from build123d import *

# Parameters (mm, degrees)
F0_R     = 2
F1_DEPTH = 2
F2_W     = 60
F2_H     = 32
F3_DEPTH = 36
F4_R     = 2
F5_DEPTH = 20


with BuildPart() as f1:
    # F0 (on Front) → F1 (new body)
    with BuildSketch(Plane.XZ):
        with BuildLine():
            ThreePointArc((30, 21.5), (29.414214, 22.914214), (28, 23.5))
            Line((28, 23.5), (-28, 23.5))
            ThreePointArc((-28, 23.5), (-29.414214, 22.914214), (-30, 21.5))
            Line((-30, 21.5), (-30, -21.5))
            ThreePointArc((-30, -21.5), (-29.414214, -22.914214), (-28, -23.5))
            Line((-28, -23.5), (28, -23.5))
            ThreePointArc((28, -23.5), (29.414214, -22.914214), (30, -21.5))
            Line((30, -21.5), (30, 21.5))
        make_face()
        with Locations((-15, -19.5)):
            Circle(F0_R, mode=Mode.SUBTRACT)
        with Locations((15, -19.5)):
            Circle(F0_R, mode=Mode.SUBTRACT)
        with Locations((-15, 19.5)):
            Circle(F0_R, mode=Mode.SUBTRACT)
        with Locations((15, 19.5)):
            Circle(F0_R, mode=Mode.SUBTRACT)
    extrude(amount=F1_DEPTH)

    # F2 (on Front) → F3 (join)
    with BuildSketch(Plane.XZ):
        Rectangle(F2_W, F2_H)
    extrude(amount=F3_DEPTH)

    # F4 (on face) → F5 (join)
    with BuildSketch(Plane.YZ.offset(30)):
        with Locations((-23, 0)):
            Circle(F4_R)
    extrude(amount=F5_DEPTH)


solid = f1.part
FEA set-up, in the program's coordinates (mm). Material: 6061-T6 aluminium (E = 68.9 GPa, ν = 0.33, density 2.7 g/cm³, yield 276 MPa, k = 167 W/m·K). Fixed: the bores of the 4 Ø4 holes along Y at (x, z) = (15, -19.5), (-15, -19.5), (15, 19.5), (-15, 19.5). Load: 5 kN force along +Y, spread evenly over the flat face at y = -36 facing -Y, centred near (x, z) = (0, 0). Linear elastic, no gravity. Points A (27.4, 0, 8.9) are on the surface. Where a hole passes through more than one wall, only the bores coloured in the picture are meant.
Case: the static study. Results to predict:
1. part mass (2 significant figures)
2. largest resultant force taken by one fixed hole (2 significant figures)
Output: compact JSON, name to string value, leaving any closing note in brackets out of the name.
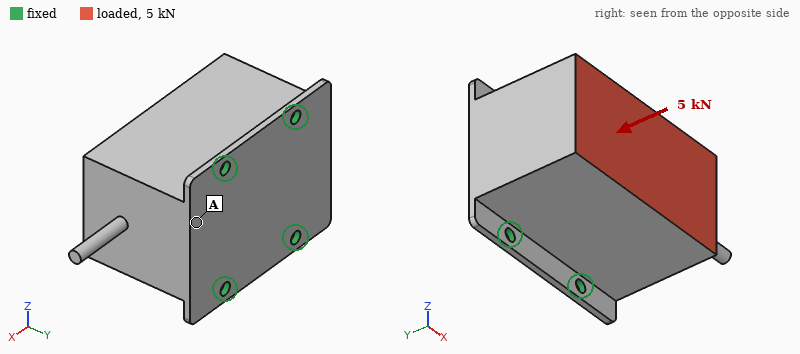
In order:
{"part mass": "190 g", "largest resultant force taken by one fixed hole": "1.4 kN"}
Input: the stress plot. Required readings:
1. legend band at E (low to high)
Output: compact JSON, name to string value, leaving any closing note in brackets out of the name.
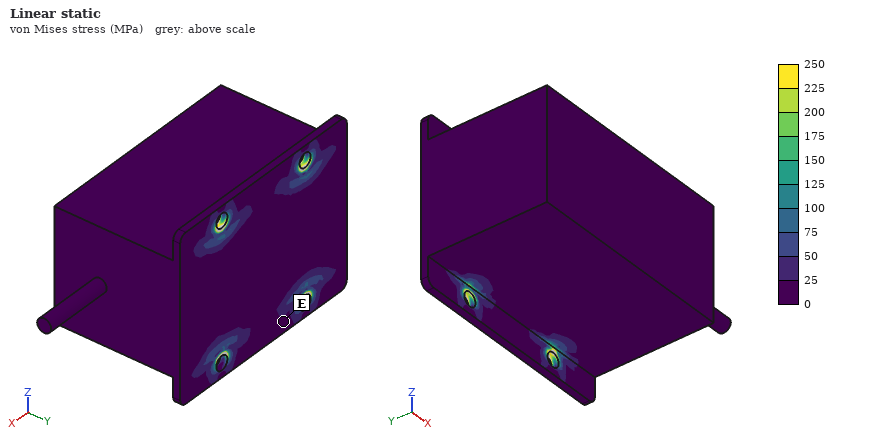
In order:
{"legend band at E": "0 to 25 MPa"}
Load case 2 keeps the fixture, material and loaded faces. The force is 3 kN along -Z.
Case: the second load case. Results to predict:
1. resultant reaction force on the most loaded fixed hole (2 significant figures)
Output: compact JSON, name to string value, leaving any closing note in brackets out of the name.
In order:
{"resultant reaction force on the most loaded fixed hole": "1.7 kN"}
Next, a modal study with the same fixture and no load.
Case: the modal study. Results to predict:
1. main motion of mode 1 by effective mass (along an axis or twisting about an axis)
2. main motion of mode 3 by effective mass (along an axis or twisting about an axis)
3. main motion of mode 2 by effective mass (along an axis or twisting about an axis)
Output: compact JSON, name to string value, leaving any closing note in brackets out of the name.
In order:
{"main motion of mode 1 by effective mass": "along X", "main motion of mode 3 by effective mass": "along Y", "main motion of mode 2 by effective mass": "along Z"}
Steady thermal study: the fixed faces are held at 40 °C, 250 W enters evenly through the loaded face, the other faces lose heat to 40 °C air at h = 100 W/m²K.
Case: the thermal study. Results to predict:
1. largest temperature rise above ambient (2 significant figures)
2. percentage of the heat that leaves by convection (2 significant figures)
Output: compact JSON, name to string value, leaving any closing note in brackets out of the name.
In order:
{"largest temperature rise above ambient": "73 K", "percentage of the heat that leaves by convection": "22 %"}
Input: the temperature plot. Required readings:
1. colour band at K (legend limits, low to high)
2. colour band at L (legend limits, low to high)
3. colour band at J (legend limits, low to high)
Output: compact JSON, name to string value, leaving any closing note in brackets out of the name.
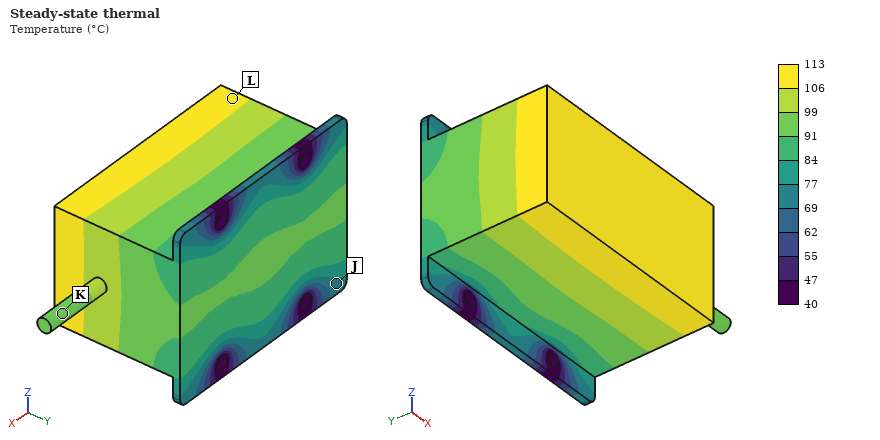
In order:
{"colour band at K": "91 to 99 °C", "colour band at L": "106 to 113 °C", "colour band at J": "69 to 77 °C"}
